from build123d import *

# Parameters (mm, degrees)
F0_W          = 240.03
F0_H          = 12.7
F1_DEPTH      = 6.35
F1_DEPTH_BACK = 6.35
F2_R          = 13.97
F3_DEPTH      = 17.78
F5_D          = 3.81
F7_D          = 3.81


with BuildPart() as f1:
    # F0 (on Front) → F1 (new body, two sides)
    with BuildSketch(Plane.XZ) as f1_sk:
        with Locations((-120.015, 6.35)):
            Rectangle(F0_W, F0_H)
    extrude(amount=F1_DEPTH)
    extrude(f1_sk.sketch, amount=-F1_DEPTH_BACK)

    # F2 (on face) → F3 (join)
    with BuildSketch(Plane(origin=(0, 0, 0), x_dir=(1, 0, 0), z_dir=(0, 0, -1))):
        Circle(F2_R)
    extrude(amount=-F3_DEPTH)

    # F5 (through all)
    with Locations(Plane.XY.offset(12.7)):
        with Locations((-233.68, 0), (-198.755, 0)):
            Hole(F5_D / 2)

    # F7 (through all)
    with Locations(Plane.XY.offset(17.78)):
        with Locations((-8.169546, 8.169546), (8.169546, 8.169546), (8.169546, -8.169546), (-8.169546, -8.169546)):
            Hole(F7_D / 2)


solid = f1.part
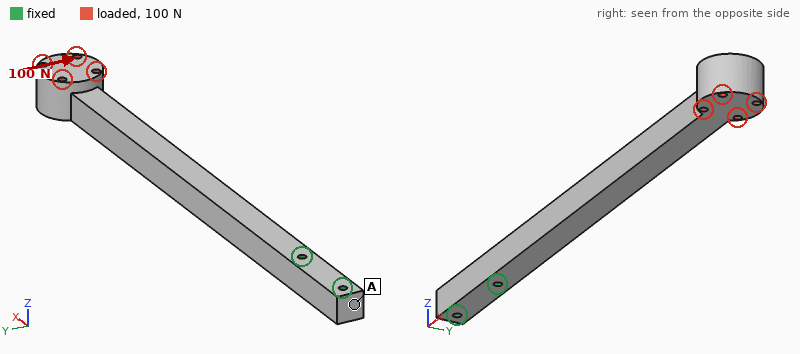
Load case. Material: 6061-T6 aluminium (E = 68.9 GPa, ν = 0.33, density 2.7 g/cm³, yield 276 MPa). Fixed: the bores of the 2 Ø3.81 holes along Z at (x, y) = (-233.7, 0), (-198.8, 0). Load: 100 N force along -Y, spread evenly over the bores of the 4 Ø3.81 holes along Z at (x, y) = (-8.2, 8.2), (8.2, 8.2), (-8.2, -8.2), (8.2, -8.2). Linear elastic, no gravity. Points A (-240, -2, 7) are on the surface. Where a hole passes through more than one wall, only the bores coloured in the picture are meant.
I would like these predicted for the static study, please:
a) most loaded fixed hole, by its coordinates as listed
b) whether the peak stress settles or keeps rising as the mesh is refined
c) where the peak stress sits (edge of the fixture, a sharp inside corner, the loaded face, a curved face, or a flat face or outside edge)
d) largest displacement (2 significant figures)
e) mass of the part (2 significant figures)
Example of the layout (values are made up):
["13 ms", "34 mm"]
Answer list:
["(-198.8, 0)", "keeps rising", "edge of the fixture", "2.1 mm", "130 g"]
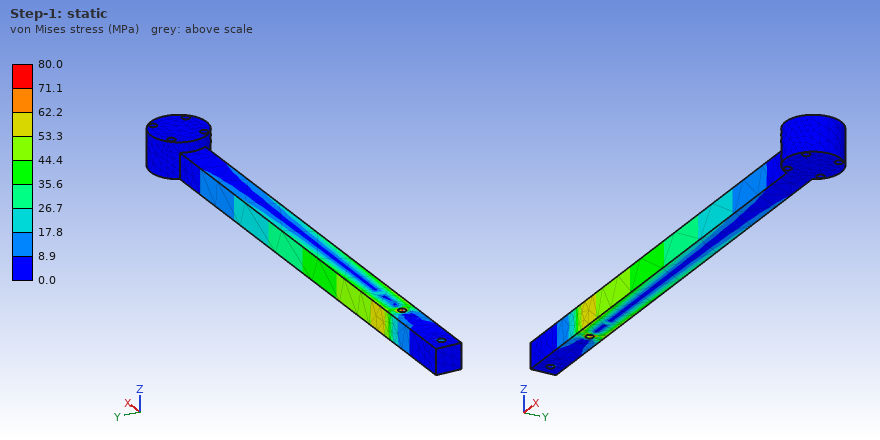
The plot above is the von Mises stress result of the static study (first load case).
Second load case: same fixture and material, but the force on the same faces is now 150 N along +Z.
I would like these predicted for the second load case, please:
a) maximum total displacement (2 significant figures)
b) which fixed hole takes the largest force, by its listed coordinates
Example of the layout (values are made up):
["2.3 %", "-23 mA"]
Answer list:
["2.9 mm", "(-198.8, 0)"]
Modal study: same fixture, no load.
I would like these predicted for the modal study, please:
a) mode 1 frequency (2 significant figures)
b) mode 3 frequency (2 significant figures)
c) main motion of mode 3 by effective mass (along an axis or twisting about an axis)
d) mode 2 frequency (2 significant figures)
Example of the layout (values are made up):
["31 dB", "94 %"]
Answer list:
["180 Hz", "1200 Hz", "along Y", "180 Hz"]
